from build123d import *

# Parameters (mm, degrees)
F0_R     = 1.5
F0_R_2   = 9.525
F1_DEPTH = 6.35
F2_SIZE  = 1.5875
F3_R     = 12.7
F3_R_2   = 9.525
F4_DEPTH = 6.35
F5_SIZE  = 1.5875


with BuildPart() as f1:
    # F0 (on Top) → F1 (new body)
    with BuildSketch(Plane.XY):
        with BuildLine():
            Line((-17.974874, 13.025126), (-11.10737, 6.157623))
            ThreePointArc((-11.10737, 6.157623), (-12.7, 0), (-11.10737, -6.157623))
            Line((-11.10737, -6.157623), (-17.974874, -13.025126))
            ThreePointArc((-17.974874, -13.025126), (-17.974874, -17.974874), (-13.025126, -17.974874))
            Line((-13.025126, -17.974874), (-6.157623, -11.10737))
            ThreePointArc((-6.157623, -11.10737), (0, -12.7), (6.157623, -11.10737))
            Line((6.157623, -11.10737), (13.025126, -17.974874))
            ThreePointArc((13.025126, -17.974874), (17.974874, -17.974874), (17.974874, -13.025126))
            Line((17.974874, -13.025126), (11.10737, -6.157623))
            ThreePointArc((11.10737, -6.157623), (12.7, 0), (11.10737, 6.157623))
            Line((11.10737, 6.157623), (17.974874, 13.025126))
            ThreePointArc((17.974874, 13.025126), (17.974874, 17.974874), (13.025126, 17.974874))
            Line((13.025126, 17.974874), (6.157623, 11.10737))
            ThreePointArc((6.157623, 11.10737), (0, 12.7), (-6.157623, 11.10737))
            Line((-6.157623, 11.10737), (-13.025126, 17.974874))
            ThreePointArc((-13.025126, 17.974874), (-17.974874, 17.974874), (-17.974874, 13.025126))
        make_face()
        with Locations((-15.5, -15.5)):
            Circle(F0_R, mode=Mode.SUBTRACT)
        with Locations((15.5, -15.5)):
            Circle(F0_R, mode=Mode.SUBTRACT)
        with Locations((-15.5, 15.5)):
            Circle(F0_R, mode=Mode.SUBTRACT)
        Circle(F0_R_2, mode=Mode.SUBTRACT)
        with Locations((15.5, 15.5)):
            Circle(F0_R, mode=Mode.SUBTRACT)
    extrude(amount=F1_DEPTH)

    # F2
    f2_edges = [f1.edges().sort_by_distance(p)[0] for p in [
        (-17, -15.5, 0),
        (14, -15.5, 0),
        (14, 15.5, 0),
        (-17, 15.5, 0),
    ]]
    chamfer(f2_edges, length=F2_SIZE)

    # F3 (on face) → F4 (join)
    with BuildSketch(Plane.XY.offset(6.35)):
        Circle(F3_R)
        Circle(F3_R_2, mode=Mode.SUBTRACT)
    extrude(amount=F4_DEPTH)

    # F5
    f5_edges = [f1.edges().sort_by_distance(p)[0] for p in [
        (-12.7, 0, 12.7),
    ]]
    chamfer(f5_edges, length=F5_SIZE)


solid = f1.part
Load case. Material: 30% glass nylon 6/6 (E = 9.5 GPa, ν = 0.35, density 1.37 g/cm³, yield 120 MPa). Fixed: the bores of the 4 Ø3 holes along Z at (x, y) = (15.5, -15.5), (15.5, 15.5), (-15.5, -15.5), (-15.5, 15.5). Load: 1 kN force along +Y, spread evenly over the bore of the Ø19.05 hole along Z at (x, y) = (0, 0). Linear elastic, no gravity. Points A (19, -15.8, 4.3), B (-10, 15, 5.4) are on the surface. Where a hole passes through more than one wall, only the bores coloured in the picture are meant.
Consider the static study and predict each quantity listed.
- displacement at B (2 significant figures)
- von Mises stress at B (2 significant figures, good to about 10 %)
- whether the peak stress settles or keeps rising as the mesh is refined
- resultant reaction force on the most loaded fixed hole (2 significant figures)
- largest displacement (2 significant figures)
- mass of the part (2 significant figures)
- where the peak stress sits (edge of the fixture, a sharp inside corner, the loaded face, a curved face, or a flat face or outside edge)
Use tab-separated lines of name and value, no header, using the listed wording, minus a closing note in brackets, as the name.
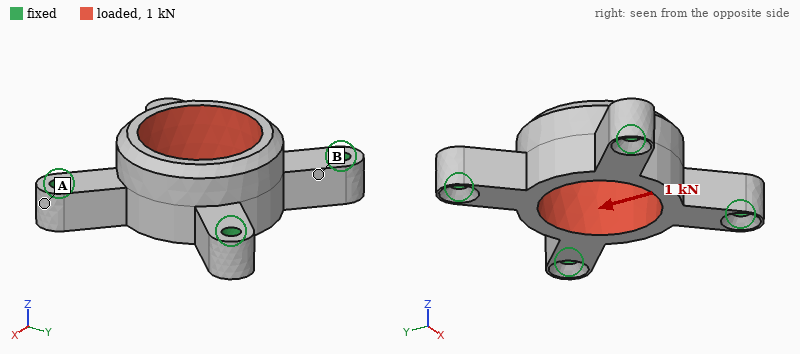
displacement at B	12 µm
von Mises stress at B	13 MPa
whether the peak stress settles or keeps rising as the mesh is refined	keeps rising
resultant reaction force on the most loaded fixed hole	300 N
largest displacement	55 µm
mass of the part	6.3 g
where the peak stress sits	edge of the fixture
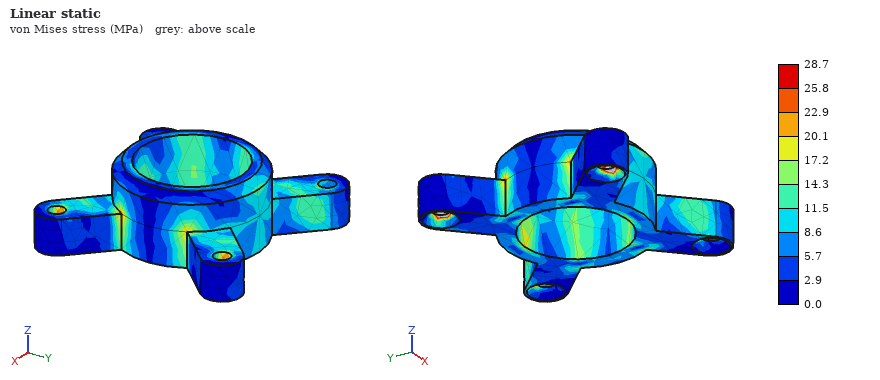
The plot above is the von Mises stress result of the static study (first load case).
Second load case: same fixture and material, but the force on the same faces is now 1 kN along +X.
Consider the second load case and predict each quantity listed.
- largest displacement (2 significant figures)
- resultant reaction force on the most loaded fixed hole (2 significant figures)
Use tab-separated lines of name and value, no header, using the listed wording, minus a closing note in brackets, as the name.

largest displacement	55 µm
resultant reaction force on the most loaded fixed hole	300 N
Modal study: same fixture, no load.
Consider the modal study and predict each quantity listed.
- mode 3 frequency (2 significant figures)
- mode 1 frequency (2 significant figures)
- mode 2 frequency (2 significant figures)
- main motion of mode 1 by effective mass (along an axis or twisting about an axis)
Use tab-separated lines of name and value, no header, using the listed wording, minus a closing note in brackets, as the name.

mode 3 frequency	13 kHz
mode 1 frequency	10000 Hz
mode 2 frequency	12 kHz
main motion of mode 1 by effective mass	along Z
